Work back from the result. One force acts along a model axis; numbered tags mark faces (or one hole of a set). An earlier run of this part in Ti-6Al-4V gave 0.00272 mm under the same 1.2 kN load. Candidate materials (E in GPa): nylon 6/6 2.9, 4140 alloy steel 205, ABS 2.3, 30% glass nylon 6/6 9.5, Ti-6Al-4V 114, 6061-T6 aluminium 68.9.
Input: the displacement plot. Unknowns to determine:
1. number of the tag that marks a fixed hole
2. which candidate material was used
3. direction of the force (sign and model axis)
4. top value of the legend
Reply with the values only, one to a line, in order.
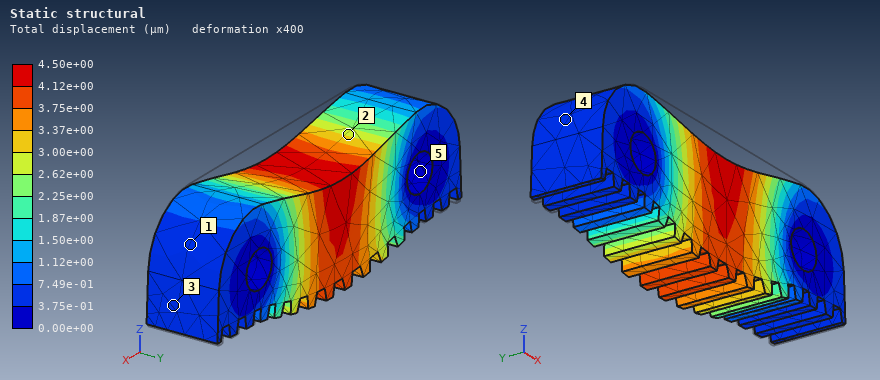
5
6061-T6 aluminium
-Z
4.50e+00 µm
